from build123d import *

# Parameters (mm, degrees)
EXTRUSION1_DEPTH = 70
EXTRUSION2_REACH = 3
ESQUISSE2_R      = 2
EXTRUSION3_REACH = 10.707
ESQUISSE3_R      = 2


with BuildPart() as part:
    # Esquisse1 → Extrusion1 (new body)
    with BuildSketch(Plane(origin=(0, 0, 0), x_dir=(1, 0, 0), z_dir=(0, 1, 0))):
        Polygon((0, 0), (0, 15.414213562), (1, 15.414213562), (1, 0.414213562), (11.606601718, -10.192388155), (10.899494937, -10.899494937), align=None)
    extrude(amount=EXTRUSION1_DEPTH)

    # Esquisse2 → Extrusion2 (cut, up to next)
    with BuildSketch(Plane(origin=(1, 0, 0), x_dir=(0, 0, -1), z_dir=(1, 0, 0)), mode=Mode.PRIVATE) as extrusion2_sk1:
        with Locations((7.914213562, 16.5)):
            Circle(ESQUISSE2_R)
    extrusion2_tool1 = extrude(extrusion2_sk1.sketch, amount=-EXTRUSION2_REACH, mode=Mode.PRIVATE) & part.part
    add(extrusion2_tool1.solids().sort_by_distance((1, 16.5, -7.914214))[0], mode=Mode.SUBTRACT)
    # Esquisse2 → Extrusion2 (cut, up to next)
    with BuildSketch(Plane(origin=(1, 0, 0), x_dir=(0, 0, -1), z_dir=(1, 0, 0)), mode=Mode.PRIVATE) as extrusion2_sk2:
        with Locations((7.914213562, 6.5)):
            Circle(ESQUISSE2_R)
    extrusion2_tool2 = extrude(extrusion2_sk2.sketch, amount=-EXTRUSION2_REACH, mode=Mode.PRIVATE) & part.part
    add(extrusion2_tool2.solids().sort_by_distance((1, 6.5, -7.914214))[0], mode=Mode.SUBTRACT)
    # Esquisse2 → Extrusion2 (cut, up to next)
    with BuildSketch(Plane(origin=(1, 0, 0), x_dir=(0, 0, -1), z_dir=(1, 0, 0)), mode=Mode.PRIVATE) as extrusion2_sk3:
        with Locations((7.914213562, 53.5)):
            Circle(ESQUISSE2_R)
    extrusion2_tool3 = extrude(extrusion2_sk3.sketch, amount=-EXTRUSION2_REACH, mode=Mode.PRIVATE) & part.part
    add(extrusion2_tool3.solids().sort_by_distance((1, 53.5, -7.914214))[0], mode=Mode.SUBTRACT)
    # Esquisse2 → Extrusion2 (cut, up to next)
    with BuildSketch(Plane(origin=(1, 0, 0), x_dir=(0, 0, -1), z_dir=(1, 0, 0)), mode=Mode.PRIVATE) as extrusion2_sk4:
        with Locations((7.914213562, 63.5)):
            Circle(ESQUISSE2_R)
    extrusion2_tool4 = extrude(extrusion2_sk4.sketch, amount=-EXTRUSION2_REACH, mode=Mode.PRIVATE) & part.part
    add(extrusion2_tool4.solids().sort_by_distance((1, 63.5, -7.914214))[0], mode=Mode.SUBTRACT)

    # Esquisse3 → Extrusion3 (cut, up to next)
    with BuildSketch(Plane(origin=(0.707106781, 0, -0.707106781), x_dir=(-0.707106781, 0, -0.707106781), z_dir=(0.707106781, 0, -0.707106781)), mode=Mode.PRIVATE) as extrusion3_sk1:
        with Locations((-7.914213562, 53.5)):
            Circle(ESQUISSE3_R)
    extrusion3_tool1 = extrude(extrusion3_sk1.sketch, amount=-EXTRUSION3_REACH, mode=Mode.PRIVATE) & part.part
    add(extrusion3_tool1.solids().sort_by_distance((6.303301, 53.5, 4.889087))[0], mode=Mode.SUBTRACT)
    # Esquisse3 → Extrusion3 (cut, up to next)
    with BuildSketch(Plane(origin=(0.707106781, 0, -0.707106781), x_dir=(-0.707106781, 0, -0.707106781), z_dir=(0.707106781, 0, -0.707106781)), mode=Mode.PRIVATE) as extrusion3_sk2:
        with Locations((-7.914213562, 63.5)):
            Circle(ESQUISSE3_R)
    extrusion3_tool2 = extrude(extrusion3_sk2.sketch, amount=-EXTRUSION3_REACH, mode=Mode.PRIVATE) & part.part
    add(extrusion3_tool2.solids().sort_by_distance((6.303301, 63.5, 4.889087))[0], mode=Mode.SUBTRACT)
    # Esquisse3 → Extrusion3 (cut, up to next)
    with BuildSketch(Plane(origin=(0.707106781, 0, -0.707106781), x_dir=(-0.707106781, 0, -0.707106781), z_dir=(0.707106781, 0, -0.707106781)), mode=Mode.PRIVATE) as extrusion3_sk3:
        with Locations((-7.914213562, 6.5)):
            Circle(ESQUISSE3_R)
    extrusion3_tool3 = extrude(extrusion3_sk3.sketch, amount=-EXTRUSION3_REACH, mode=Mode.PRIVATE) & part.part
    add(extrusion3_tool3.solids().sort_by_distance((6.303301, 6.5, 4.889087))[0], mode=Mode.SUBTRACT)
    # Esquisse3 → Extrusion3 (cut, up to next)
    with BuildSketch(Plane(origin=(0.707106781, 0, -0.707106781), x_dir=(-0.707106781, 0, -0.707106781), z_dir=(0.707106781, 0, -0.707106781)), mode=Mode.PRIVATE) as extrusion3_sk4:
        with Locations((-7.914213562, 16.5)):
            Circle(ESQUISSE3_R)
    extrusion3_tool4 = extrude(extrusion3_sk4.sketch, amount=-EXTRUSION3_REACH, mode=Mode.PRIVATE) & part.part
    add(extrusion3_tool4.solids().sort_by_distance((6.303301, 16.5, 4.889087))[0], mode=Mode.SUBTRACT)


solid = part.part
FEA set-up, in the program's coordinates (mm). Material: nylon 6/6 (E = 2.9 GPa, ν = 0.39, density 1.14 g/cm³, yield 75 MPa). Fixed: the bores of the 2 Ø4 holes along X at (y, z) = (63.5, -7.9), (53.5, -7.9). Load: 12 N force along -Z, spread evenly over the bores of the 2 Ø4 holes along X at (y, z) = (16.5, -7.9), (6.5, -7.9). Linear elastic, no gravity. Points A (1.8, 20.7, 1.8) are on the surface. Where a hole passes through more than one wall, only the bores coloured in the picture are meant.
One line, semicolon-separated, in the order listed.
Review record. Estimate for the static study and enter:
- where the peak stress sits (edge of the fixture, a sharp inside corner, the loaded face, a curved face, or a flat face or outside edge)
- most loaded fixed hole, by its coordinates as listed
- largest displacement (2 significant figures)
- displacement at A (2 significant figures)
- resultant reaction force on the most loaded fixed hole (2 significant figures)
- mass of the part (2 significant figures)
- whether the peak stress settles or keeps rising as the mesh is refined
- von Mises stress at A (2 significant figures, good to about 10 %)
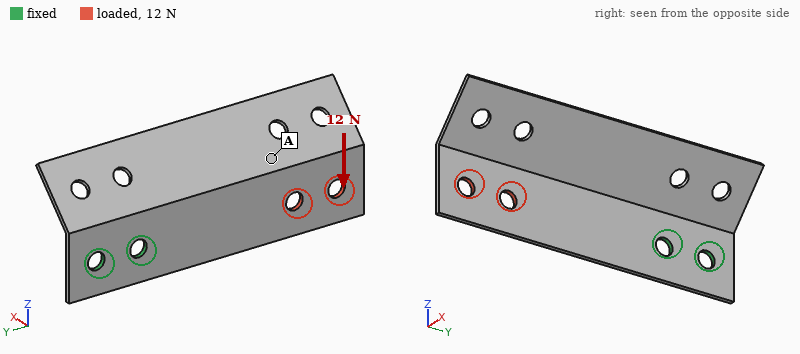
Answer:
edge of the fixture; (53.5, -7.9); 0.85 mm; 0.44 mm; 41 N; 2.3 g; keeps rising; 1.6 MPa
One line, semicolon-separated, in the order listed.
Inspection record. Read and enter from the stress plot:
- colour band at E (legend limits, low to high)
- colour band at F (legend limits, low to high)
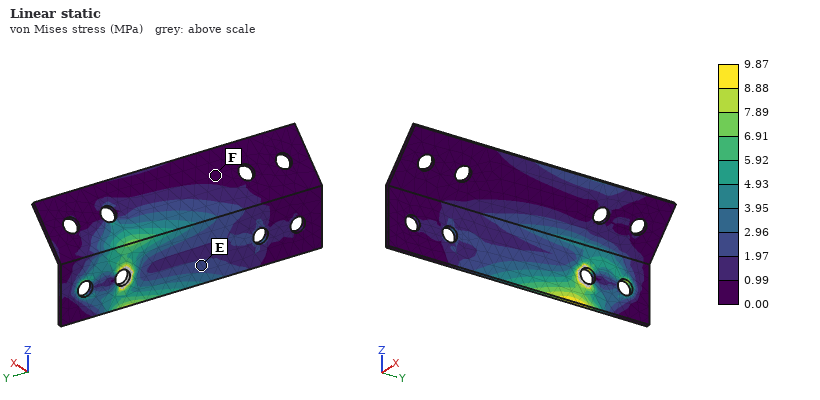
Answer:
1.97 to 2.96 MPa; 0.00 to 0.99 MPa
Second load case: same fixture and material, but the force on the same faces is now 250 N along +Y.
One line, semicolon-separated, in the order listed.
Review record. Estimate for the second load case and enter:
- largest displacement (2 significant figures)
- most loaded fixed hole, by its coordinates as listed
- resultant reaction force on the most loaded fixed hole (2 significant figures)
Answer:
0.48 mm; (53.5, -7.9); 200 N
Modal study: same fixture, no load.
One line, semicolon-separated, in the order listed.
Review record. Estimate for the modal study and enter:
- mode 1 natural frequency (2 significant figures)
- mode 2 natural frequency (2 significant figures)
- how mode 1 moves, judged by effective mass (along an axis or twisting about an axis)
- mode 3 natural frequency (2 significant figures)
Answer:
220 Hz; 320 Hz; along X; 680 Hz
